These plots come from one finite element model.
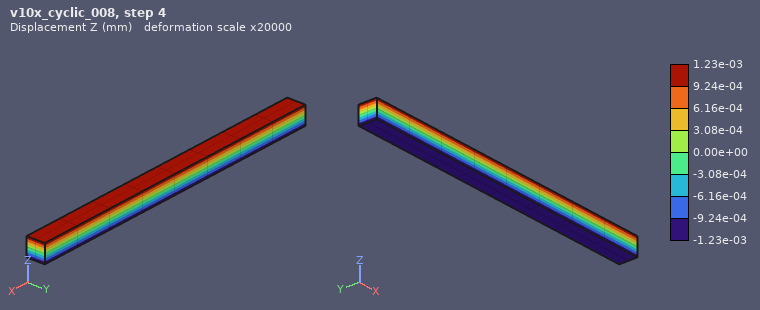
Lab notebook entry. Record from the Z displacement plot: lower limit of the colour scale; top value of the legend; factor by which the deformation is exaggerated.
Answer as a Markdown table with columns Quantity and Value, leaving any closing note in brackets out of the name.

| Quantity | Value |
|---|---|
| lower limit of the colour scale | -1.23e-03 mm |
| top value of the legend | 1.23e-03 mm |
| factor by which the deformation is exaggerated | 20000 |
